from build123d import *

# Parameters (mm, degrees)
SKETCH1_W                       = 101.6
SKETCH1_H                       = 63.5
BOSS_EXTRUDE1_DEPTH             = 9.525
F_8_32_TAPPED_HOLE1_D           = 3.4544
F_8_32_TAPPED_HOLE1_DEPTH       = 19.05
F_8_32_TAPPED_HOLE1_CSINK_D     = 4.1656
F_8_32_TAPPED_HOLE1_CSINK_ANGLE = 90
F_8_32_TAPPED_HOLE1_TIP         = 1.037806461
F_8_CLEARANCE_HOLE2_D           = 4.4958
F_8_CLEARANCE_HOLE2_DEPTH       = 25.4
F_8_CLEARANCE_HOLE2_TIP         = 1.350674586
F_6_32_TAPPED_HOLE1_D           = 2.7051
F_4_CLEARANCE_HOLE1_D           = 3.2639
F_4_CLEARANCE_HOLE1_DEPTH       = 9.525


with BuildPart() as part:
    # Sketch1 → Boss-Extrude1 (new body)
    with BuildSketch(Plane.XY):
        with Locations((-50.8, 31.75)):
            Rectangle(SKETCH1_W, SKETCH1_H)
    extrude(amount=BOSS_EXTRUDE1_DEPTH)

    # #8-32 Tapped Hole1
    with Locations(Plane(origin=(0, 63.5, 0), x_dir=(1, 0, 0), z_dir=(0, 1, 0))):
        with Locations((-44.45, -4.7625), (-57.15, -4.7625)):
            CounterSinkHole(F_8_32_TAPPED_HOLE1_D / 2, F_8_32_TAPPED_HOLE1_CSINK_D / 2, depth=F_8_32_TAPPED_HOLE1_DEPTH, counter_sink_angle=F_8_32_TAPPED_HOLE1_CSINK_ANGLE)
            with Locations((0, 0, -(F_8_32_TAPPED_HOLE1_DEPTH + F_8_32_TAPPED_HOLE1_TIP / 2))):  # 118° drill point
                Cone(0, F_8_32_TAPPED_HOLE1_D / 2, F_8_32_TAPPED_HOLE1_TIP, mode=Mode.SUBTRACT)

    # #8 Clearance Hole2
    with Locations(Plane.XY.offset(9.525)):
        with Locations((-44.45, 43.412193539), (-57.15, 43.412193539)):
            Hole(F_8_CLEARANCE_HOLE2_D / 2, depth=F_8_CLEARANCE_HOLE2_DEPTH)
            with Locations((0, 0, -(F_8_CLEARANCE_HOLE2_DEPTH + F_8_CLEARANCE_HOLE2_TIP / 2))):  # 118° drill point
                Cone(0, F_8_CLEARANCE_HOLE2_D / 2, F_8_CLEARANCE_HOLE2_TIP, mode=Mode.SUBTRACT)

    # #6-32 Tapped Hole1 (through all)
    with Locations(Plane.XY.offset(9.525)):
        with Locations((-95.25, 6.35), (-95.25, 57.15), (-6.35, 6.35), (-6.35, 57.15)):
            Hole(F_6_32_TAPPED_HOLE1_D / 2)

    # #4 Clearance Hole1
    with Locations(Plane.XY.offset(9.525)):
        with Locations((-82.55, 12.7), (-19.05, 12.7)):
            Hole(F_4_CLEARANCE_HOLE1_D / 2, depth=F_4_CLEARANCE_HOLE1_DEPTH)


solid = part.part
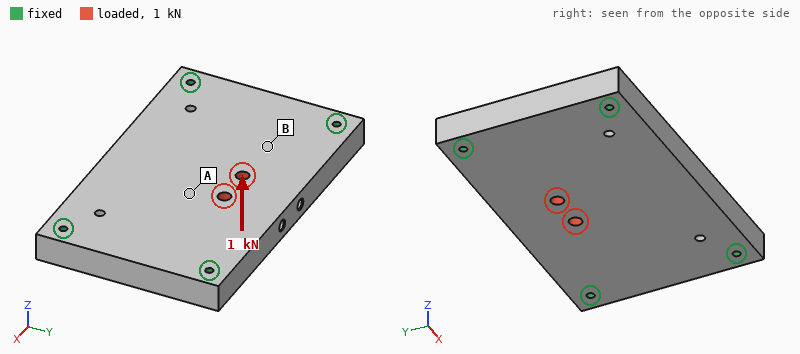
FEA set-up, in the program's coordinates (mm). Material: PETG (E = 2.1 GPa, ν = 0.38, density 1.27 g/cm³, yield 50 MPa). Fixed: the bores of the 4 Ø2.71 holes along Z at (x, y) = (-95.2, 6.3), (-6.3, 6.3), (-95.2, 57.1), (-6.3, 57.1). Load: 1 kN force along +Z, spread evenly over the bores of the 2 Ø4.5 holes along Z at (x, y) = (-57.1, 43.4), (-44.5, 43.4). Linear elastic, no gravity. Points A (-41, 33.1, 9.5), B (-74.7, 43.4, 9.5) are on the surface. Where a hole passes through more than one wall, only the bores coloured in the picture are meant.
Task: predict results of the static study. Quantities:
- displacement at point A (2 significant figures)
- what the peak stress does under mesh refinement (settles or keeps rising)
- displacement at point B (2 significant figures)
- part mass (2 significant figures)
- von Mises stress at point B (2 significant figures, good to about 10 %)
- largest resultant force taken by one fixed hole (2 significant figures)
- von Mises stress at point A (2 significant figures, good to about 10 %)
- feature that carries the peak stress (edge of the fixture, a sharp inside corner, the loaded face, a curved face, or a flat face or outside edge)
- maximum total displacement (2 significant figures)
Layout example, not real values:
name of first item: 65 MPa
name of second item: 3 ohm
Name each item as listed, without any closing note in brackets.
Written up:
displacement at point A: 0.61 mm
what the peak stress does under mesh refinement: keeps rising
displacement at point B: 0.44 mm
part mass: 77 g
von Mises stress at point B: 4.6 MPa
largest resultant force taken by one fixed hole: 360 N
von Mises stress at point A: 10 MPa
feature that carries the peak stress: edge of the fixture
maximum total displacement: 0.83 mm
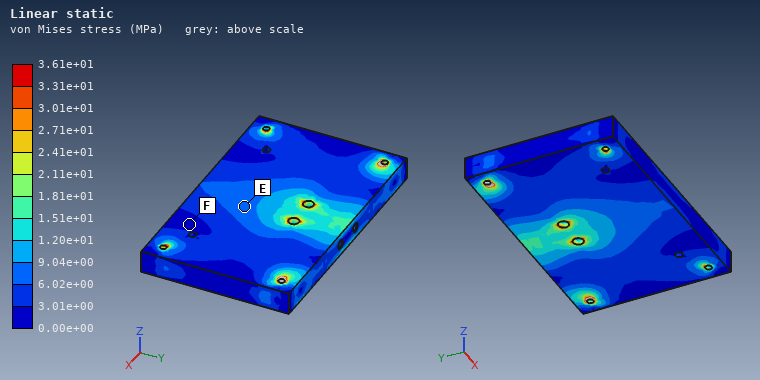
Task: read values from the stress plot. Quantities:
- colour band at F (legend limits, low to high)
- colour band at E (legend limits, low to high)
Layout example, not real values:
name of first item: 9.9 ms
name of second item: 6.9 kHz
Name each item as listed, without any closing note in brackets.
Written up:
colour band at F: 0.00e+00 to 3.01e+00 MPa
colour band at E: 6.02e+00 to 9.04e+00 MPa
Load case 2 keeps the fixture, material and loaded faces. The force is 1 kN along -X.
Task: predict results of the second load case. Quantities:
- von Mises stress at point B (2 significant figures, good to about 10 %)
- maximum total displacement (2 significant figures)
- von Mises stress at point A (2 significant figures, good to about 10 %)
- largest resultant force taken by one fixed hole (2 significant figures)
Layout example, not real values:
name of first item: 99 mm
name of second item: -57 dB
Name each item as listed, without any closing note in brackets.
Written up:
von Mises stress at point B: 1.4 MPa
maximum total displacement: 54 µm
von Mises stress at point A: 1.3 MPa
largest resultant force taken by one fixed hole: 310 N
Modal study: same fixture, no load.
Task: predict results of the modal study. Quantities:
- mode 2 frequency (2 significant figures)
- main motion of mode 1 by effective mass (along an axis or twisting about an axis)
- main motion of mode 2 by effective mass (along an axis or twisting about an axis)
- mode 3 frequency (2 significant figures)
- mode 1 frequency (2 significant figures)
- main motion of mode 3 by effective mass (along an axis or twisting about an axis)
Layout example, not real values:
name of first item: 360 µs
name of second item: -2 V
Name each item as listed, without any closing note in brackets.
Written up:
mode 2 frequency: 1800 Hz
main motion of mode 1 by effective mass: along Z
main motion of mode 2 by effective mass: twisting about X
mode 3 frequency: 2900 Hz
mode 1 frequency: 1100 Hz
main motion of mode 3 by effective mass: twisting about Y
